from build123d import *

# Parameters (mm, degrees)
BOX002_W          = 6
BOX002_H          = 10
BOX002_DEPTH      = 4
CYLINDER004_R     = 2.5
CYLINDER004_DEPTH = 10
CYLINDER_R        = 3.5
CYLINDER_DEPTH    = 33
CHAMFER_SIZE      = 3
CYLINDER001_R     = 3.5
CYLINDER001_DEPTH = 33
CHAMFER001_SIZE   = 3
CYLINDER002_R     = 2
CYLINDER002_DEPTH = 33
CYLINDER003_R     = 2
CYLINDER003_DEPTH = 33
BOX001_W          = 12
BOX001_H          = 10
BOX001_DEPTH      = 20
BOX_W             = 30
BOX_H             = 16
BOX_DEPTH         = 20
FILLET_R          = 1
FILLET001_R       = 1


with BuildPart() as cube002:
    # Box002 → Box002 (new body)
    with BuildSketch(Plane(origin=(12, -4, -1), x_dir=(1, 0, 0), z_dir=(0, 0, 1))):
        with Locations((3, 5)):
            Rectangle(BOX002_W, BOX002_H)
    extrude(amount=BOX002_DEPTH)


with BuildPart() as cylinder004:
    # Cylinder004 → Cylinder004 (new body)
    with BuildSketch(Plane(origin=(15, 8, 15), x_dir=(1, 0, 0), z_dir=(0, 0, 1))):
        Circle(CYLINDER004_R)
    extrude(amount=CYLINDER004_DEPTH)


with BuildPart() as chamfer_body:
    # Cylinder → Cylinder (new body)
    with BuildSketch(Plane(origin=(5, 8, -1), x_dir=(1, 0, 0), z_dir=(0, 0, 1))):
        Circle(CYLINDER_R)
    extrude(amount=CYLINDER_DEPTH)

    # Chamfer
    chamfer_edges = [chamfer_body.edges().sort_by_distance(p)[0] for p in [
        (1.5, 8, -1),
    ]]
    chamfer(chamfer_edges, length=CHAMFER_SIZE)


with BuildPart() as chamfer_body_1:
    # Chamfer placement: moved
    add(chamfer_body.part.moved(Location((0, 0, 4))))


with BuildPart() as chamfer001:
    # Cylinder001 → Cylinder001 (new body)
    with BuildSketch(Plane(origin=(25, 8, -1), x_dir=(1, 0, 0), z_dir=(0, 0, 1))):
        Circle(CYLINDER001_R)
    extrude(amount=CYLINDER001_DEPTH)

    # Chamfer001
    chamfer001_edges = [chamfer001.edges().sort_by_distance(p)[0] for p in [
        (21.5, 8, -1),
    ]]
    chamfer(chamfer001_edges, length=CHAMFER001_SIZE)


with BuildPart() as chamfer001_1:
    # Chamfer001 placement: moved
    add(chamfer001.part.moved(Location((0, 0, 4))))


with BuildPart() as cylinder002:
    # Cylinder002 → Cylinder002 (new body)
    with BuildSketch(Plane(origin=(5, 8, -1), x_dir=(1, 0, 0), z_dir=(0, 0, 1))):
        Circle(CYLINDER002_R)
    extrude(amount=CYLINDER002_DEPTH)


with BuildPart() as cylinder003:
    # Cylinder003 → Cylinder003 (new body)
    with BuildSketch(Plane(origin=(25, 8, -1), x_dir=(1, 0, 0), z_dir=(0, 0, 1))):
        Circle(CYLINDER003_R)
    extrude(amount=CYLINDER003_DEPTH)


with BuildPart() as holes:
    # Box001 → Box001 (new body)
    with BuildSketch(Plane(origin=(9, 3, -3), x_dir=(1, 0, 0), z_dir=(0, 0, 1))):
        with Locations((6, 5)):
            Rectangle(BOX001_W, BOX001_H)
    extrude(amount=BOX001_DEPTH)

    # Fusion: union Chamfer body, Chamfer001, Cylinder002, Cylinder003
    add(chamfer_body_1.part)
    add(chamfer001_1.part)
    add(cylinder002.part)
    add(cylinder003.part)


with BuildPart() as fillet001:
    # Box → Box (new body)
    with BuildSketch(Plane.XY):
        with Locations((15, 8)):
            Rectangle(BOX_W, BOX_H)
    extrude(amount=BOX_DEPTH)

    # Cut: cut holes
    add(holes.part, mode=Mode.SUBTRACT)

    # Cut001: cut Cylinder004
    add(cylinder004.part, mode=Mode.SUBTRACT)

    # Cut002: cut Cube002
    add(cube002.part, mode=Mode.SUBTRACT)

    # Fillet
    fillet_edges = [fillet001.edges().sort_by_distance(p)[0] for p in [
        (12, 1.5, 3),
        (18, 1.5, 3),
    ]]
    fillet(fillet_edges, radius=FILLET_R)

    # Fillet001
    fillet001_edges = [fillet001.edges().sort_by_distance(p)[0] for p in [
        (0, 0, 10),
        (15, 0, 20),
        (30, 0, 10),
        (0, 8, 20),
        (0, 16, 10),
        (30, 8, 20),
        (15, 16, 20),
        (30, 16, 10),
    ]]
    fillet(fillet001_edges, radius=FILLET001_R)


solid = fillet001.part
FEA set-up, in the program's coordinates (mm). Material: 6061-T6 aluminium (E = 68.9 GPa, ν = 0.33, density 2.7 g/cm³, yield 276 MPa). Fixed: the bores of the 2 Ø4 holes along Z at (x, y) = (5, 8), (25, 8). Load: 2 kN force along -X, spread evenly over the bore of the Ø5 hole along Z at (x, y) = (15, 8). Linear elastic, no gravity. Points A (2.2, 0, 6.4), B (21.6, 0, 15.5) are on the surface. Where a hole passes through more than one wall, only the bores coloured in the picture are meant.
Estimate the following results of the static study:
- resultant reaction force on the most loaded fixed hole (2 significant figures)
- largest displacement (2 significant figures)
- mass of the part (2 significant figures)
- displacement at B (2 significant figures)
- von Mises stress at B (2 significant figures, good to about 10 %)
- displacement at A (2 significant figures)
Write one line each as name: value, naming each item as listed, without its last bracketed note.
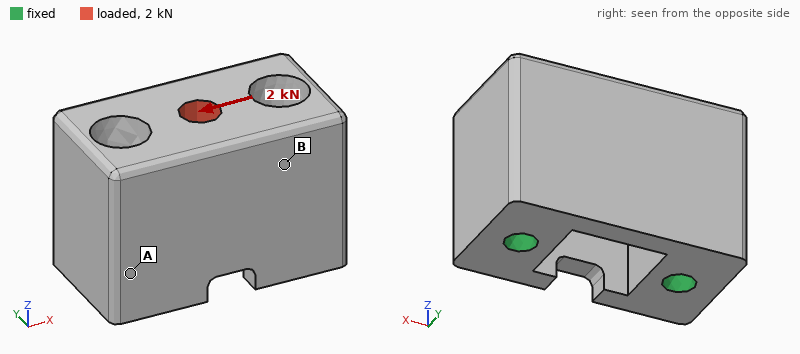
resultant reaction force on the most loaded fixed hole: 1.6 kN
largest displacement: 20 µm
mass of the part: 17 g
displacement at B: 12 µm
von Mises stress at B: 15 MPa
displacement at A: 7.1 µm
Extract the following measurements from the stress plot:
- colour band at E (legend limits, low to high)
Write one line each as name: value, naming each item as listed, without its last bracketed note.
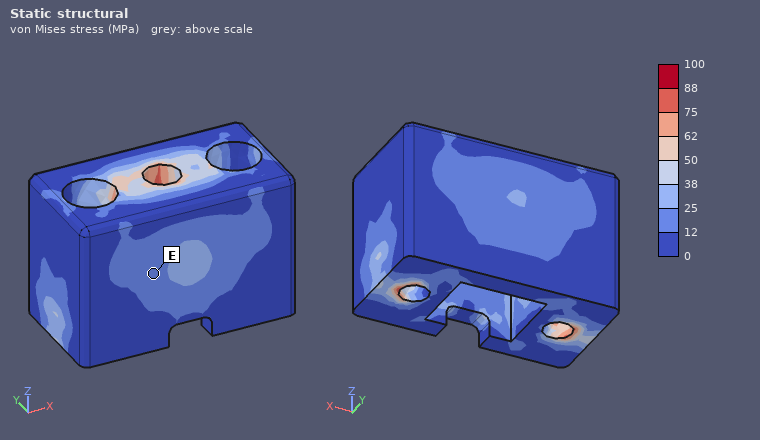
colour band at E: 12 to 25 MPa
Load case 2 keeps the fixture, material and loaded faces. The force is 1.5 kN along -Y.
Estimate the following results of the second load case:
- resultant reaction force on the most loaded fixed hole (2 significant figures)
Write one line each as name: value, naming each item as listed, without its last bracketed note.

resultant reaction force on the most loaded fixed hole: 750 N
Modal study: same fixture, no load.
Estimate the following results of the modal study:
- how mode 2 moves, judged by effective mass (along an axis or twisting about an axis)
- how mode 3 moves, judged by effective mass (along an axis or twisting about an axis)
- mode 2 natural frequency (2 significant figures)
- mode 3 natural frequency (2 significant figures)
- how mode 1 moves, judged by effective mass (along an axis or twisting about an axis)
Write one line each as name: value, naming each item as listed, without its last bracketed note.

how mode 2 moves, judged by effective mass: along X
how mode 3 moves, judged by effective mass: twisting about Z
mode 2 natural frequency: 21 kHz
mode 3 natural frequency: 23 kHz
how mode 1 moves, judged by effective mass: along Y
